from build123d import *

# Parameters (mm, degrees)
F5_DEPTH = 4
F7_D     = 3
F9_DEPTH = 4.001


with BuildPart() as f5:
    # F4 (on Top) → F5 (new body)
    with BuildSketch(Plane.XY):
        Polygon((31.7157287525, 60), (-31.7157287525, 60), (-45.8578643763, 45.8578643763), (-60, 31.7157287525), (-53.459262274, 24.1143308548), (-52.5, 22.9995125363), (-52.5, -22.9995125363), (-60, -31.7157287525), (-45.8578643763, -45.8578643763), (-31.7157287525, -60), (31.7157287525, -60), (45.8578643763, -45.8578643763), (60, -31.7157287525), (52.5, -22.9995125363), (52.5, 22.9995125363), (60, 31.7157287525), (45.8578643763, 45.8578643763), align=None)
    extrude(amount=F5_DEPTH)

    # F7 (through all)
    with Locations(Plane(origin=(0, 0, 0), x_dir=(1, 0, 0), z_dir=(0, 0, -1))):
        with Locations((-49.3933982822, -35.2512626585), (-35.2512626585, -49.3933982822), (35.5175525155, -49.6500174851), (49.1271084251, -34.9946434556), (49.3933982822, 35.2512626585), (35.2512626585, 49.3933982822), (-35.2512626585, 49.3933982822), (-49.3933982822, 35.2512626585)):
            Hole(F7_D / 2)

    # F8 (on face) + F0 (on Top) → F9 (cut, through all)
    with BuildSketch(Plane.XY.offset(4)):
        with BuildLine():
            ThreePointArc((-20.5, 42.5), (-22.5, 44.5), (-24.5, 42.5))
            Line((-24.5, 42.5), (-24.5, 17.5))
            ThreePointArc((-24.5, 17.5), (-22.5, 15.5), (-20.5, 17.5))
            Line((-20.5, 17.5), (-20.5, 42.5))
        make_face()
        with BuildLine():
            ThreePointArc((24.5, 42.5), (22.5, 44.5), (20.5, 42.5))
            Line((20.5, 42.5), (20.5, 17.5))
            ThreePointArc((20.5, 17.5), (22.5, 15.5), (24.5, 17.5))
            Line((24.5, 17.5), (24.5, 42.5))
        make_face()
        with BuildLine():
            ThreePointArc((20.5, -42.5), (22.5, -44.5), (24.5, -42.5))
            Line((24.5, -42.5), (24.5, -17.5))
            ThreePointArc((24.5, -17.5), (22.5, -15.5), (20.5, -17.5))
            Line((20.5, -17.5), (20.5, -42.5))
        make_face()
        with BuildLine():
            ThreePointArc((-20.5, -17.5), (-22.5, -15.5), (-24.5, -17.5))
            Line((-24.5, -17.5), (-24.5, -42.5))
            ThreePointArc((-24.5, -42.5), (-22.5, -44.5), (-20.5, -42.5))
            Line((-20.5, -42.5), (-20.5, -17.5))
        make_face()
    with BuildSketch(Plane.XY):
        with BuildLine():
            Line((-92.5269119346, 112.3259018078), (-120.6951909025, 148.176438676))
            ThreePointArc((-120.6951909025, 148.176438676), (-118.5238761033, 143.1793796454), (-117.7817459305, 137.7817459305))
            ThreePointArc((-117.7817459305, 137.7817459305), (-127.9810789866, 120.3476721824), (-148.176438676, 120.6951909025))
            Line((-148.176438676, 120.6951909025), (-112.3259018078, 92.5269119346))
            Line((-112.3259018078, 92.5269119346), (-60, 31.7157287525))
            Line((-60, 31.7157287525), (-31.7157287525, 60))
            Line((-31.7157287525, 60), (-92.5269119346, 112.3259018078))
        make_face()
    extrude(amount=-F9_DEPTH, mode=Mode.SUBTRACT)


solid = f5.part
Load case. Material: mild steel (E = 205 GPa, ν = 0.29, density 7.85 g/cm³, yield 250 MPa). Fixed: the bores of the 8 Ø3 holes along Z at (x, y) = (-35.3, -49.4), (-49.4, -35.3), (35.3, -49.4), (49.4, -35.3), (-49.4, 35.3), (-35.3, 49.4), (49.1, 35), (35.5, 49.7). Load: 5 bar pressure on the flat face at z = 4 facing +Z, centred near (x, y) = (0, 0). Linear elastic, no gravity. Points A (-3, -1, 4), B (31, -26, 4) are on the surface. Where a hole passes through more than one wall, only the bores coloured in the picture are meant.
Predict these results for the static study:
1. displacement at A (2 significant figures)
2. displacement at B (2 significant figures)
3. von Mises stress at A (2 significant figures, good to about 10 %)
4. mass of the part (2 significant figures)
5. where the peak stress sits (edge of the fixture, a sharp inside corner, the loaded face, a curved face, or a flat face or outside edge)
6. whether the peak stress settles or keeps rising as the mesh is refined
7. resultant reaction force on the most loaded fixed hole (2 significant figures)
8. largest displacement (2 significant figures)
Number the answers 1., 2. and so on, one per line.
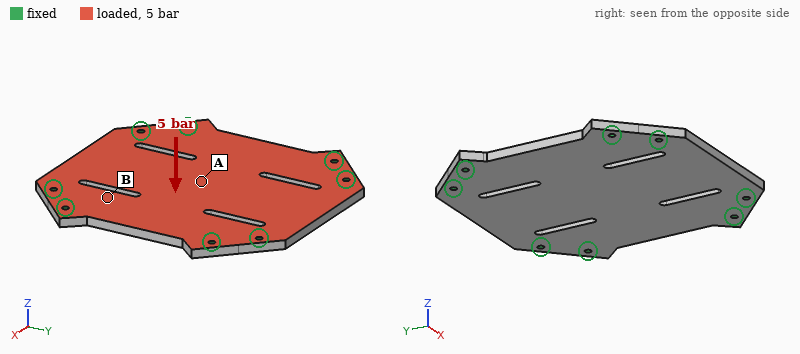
1. 0.15 mm
2. 0.056 mm
3. 66 MPa
4. 360 g
5. edge of the fixture
6. keeps rising
7. 800 N
8. 0.15 mm
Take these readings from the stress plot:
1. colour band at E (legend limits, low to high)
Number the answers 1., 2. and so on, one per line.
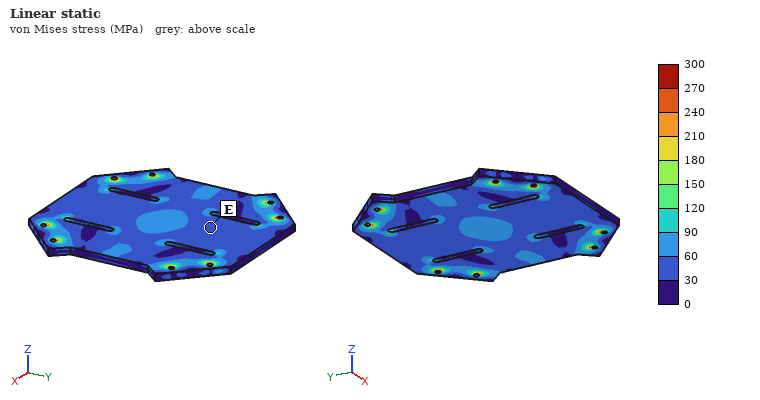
1. 30 to 60 MPa
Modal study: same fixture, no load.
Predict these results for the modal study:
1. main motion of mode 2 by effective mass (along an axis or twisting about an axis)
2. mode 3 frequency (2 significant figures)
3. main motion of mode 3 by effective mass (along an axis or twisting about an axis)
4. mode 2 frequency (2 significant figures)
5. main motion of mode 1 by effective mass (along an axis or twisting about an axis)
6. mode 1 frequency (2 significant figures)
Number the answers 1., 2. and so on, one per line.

1. twisting about X
2. 3800 Hz
3. twisting about Y
4. 3600 Hz
5. along Z
6. 2000 Hz
